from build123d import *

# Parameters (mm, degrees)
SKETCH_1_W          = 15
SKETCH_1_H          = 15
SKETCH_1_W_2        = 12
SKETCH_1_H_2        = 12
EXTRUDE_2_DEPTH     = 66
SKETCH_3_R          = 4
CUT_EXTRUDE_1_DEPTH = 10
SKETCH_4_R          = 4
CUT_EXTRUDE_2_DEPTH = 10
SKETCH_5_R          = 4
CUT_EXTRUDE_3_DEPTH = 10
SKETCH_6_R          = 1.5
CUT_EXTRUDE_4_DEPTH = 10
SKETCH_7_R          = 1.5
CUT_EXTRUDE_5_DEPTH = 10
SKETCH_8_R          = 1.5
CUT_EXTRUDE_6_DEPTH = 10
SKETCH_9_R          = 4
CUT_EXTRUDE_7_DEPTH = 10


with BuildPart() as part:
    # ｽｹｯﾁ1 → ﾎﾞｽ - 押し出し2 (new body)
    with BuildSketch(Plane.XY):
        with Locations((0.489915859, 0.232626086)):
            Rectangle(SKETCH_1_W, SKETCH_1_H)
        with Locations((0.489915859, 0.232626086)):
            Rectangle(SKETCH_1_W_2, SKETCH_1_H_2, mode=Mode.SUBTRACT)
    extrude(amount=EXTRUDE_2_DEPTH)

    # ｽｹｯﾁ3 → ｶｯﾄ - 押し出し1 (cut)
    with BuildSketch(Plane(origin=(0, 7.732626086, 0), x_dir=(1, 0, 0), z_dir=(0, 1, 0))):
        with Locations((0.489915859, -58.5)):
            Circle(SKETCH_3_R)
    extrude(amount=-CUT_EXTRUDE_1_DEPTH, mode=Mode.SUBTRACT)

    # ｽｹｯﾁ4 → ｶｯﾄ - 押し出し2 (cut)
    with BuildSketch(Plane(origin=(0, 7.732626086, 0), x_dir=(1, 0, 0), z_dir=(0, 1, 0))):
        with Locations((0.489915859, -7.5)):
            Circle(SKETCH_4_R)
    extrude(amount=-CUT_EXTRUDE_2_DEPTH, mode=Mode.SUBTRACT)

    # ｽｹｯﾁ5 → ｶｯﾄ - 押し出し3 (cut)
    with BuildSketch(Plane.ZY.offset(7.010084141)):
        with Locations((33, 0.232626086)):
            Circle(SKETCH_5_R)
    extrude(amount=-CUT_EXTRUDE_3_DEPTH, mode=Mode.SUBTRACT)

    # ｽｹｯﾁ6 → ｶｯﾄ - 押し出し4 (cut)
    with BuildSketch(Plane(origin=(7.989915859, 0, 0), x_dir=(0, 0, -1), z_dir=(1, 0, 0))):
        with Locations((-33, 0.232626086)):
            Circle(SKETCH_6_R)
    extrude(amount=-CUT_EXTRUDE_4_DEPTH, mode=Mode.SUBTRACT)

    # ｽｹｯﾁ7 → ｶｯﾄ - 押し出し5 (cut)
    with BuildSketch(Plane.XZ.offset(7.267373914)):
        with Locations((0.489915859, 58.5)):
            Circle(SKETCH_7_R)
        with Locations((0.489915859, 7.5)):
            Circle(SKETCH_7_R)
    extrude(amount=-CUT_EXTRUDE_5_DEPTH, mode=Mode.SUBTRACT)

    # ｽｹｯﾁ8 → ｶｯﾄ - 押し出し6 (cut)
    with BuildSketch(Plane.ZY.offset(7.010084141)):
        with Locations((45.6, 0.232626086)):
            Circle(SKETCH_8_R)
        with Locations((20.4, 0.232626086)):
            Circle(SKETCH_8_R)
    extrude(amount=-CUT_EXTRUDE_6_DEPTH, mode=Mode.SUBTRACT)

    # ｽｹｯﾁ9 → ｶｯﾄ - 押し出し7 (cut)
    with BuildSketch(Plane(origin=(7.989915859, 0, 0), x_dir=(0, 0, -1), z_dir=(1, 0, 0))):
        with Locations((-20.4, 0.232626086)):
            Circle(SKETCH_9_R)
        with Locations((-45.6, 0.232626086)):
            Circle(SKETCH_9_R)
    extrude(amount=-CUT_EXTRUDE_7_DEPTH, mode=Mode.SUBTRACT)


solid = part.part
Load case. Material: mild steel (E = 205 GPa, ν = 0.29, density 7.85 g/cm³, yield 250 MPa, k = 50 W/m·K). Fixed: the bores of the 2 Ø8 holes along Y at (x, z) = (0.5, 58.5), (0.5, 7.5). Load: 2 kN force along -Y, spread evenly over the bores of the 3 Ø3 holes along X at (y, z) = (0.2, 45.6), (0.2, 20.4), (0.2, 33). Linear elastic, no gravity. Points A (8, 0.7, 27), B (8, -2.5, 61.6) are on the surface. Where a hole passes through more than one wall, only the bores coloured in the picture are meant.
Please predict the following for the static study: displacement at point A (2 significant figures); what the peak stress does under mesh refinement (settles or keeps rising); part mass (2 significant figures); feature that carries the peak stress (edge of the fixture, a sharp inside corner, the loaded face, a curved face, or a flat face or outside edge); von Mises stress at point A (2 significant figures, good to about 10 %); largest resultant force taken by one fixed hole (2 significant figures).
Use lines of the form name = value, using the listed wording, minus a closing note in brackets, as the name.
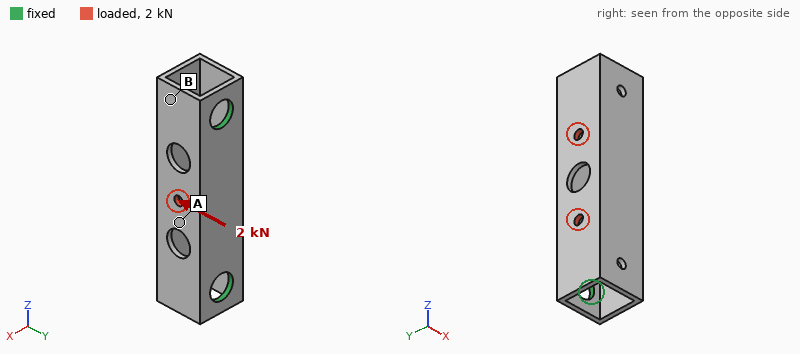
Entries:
displacement at point A = 15 µm
what the peak stress does under mesh refinement = keeps rising
part mass = 39 g
feature that carries the peak stress = edge of the fixture
von Mises stress at point A = 58 MPa
largest resultant force taken by one fixed hole = 1.3 kN
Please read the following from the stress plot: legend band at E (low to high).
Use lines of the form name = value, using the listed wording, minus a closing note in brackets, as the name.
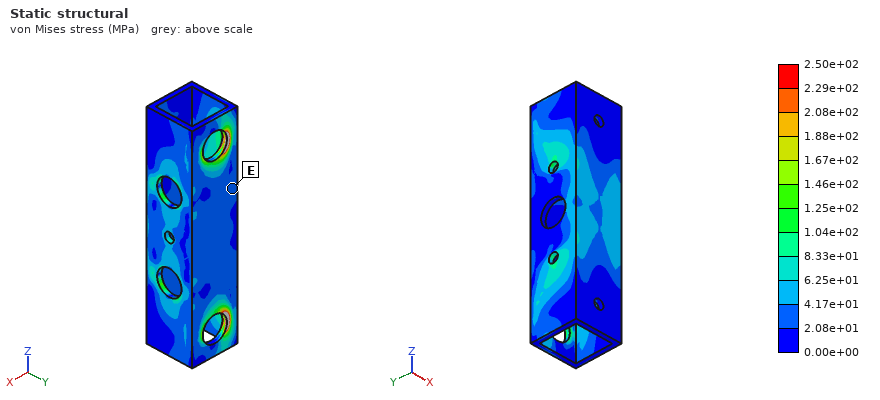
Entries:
legend band at E = 2.08e+01 to 4.17e+01 MPa
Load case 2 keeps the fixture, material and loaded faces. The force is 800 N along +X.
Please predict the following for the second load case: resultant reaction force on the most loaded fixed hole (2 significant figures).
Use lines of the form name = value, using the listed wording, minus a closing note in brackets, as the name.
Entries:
resultant reaction force on the most loaded fixed hole = 400 N
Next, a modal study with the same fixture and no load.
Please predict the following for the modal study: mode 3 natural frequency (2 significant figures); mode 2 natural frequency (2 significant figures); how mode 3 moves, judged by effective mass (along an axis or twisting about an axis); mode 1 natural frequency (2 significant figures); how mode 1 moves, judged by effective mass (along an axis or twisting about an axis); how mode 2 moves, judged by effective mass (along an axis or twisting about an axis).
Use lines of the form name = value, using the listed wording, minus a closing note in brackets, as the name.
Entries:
mode 3 natural frequency = 11 kHz
mode 2 natural frequency = 9900 Hz
how mode 3 moves, judged by effective mass = along Y
mode 1 natural frequency = 3900 Hz
how mode 1 moves, judged by effective mass = along X
how mode 2 moves, judged by effective mass = twisting about Y
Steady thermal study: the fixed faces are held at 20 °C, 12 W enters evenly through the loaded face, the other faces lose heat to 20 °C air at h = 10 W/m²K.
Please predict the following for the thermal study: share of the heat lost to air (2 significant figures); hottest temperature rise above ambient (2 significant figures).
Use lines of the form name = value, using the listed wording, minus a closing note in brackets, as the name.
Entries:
share of the heat lost to air = 12 %
hottest temperature rise above ambient = 47 K
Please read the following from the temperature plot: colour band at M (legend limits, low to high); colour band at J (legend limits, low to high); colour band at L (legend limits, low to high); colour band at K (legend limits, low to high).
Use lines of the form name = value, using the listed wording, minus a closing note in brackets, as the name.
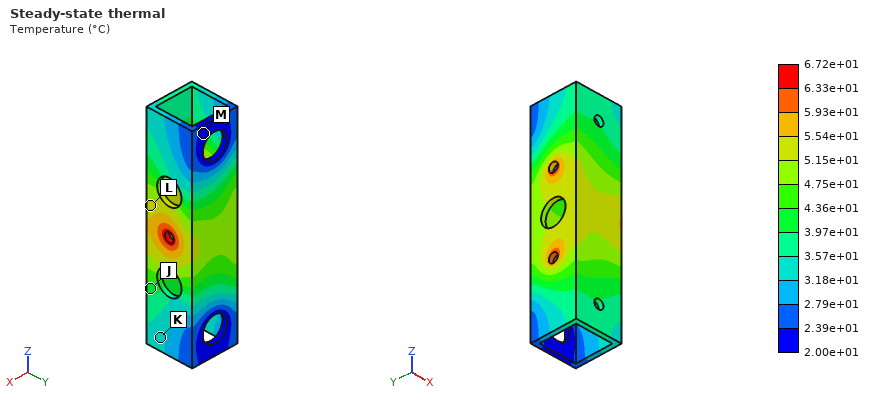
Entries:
colour band at M = 2.00e+01 to 2.39e+01 °C
colour band at J = 3.97e+01 to 4.36e+01 °C
colour band at L = 5.15e+01 to 5.54e+01 °C
colour band at K = 3.18e+01 to 3.57e+01 °C
